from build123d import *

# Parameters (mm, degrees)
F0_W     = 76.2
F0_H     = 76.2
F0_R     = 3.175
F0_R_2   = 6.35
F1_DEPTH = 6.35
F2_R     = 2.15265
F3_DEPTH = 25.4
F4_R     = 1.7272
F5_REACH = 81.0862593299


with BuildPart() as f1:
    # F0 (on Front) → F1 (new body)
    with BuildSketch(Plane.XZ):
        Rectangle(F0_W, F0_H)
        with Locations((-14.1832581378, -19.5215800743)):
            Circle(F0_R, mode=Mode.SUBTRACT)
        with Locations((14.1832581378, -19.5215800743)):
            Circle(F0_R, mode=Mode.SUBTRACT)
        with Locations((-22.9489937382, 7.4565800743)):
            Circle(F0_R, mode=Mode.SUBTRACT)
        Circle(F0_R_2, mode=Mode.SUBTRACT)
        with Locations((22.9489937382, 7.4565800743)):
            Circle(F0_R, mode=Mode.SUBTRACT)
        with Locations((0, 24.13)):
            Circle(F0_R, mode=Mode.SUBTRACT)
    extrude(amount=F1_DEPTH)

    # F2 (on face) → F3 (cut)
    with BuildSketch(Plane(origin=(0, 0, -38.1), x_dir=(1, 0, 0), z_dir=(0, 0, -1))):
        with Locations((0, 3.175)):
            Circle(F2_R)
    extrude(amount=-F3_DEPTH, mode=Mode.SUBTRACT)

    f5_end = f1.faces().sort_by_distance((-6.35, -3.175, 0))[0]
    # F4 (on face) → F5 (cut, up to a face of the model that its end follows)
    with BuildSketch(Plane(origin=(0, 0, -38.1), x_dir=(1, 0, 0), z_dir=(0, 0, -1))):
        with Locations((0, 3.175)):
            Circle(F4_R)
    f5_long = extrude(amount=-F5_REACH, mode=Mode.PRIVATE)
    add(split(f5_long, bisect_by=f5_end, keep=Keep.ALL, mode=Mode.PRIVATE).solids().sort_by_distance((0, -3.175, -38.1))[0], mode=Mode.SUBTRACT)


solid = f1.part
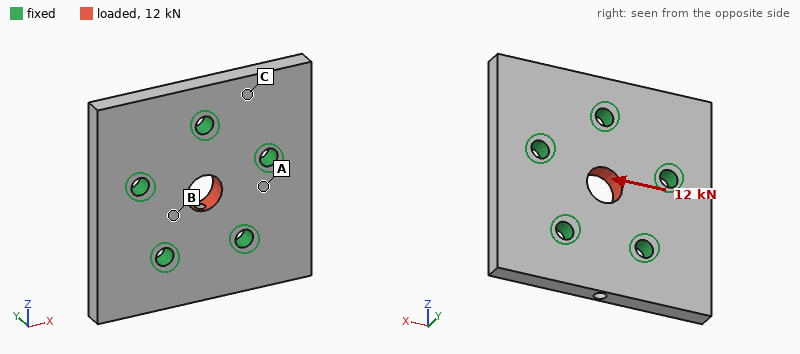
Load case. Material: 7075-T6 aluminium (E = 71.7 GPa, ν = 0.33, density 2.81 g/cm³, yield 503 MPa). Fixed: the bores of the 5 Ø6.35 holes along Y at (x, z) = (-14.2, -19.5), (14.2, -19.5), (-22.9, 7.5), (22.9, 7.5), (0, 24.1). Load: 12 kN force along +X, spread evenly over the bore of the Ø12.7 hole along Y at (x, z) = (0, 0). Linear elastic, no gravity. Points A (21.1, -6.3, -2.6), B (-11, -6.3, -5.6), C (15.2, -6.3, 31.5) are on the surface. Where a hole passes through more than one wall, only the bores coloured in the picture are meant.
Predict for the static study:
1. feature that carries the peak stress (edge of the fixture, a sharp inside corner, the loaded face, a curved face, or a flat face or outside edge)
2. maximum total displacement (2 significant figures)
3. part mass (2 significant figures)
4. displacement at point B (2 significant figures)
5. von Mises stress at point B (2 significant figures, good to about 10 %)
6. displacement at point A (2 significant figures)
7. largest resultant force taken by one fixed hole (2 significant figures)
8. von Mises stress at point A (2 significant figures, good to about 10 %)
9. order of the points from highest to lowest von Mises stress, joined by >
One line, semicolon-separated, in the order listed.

a curved face; 10 µm; 97 g; 6.3 µm; 30 MPa; 3.7 µm; 3.6 kN; 15 MPa; B > A > C
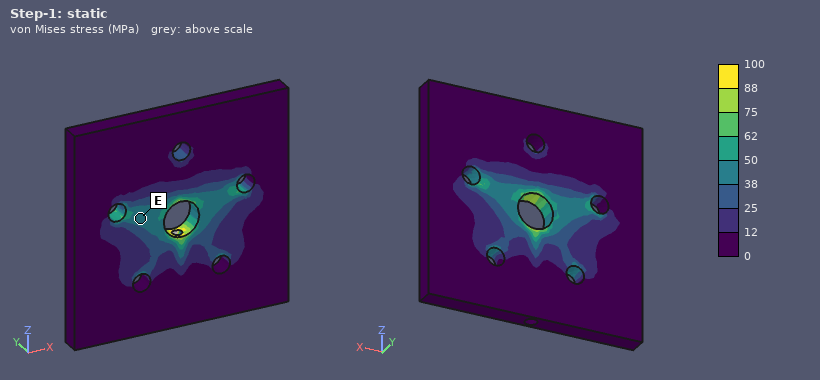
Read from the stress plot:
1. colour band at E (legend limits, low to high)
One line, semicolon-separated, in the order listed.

38 to 50 MPa
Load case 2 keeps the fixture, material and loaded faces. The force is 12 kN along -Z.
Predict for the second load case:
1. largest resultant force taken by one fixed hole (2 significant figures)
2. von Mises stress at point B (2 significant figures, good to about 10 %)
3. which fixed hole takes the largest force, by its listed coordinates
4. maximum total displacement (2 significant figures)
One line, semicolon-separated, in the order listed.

3.7 kN; 29 MPa; (0, 24.1); 10 µm
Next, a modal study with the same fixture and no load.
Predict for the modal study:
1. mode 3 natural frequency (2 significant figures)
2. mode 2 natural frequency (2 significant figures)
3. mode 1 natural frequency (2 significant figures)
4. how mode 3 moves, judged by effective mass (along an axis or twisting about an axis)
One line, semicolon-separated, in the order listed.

9200 Hz; 8100 Hz; 7800 Hz; twisting about Z
